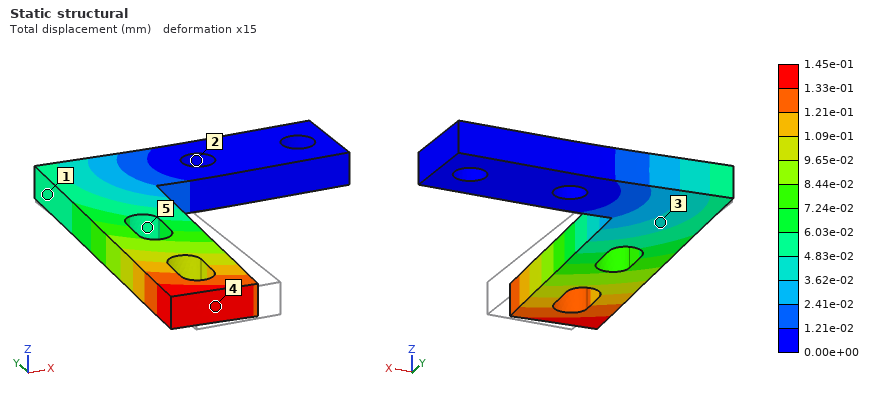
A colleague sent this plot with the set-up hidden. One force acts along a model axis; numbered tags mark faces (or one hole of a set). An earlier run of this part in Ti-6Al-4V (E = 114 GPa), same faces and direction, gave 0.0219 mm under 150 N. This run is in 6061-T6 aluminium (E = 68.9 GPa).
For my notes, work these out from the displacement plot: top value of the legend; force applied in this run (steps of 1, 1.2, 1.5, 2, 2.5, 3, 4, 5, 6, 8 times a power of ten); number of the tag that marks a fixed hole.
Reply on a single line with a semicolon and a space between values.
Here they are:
1.45e-01 mm; 600 N; 2
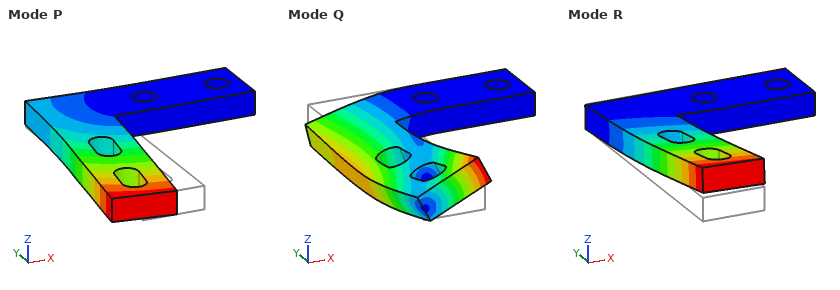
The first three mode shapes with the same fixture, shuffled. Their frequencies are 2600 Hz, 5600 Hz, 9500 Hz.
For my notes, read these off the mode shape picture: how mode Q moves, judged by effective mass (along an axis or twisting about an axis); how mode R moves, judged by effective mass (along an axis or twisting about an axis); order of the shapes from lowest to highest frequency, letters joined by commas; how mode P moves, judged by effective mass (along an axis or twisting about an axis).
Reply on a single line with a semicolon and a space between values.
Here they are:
along Z; along Z; R, P, Q; along X
